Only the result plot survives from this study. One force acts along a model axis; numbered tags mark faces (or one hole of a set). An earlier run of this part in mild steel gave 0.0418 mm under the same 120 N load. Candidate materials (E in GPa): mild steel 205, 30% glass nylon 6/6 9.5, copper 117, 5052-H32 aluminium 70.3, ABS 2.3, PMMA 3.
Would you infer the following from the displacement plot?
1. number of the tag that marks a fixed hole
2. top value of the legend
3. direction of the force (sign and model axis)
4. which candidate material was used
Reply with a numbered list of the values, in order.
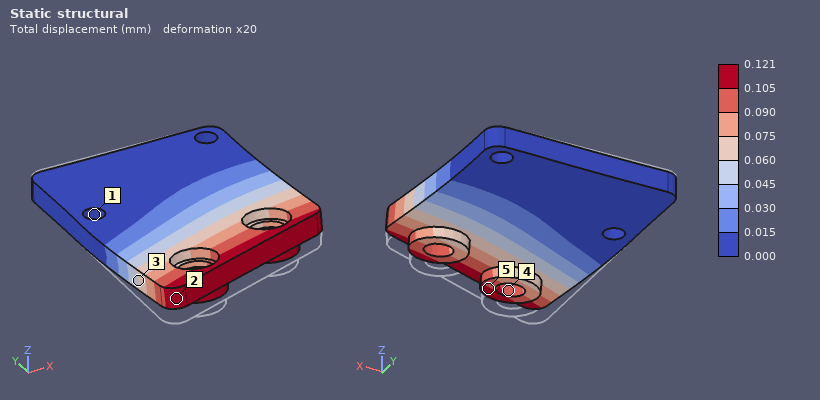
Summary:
1. 1
2. 0.121 mm
3. +Z
4. 5052-H32 aluminium
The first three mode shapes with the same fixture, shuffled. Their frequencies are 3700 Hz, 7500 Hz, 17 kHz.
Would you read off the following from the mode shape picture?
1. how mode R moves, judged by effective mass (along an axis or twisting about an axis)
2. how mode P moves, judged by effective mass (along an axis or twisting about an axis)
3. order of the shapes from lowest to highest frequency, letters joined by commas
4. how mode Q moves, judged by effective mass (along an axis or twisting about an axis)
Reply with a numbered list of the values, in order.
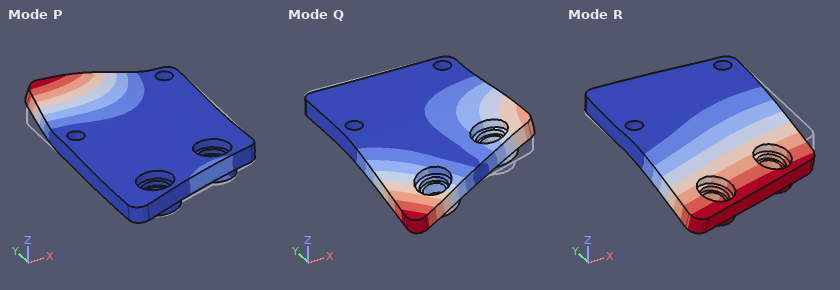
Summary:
1. along Z
2. along Z
3. R, Q, P
4. twisting about Y
